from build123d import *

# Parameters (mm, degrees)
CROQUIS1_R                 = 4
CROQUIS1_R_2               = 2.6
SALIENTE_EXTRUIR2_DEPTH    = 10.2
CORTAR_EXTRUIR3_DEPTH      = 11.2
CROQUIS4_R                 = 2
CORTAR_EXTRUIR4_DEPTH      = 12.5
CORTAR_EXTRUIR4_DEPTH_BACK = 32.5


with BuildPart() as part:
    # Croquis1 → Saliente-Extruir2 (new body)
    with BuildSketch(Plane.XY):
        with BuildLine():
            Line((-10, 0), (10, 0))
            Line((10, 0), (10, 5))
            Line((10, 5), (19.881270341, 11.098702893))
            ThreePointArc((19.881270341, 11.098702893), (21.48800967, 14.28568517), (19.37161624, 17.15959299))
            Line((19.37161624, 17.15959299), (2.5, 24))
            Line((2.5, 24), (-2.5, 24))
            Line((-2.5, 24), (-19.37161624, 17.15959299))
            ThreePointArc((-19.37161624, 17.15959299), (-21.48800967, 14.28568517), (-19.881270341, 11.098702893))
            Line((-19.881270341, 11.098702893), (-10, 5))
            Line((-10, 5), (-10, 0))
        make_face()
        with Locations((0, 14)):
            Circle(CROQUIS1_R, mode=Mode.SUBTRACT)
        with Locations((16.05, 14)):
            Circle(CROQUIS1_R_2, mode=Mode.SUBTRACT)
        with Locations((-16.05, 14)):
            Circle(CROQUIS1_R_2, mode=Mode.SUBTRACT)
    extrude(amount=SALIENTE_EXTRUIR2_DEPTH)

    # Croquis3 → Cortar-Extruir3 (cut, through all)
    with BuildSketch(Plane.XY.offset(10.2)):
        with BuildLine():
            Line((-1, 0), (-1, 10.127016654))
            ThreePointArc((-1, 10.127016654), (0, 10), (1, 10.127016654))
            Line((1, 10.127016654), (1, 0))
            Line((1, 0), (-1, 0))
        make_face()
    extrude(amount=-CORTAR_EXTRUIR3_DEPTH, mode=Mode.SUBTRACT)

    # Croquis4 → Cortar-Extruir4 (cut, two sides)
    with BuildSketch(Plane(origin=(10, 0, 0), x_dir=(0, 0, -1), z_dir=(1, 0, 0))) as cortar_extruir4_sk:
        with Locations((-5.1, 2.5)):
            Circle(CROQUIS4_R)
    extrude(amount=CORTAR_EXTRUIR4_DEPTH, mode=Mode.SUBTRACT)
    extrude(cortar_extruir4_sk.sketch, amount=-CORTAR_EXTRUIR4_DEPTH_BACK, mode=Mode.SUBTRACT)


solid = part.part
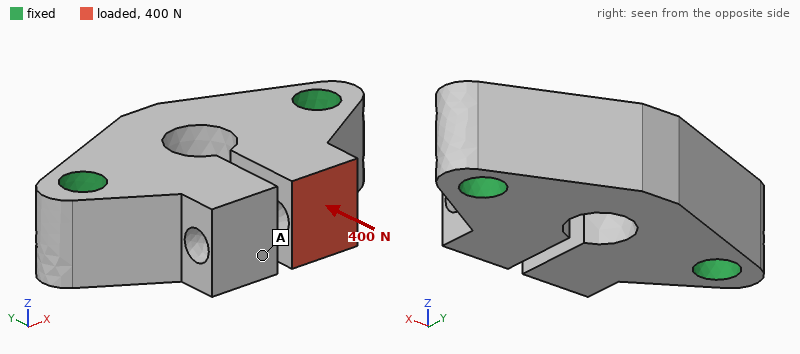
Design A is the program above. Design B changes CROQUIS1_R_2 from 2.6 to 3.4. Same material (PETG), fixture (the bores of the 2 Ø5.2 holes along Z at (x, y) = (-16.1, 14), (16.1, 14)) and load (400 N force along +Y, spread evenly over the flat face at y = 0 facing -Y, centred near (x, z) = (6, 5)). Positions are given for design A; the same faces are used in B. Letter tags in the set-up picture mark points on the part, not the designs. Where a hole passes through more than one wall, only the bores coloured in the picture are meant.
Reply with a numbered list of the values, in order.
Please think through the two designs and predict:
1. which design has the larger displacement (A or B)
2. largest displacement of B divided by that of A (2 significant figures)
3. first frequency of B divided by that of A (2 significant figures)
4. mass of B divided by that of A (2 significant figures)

1. A
2. 0.89
3. 1.1
4. 0.95
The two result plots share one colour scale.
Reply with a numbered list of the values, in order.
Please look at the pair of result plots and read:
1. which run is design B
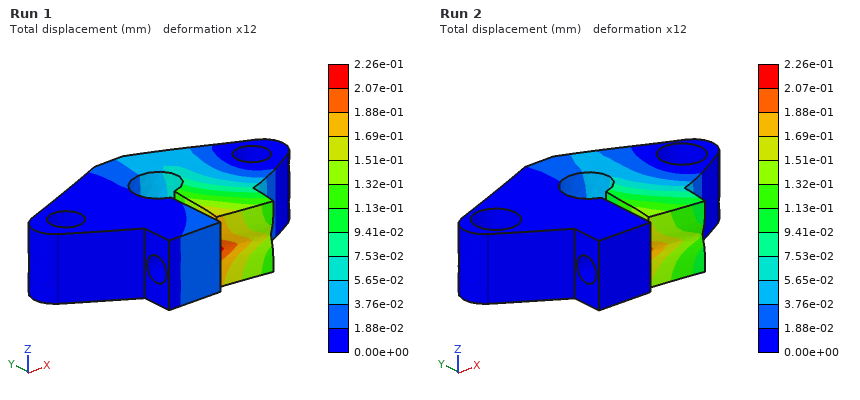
1. Run 2
